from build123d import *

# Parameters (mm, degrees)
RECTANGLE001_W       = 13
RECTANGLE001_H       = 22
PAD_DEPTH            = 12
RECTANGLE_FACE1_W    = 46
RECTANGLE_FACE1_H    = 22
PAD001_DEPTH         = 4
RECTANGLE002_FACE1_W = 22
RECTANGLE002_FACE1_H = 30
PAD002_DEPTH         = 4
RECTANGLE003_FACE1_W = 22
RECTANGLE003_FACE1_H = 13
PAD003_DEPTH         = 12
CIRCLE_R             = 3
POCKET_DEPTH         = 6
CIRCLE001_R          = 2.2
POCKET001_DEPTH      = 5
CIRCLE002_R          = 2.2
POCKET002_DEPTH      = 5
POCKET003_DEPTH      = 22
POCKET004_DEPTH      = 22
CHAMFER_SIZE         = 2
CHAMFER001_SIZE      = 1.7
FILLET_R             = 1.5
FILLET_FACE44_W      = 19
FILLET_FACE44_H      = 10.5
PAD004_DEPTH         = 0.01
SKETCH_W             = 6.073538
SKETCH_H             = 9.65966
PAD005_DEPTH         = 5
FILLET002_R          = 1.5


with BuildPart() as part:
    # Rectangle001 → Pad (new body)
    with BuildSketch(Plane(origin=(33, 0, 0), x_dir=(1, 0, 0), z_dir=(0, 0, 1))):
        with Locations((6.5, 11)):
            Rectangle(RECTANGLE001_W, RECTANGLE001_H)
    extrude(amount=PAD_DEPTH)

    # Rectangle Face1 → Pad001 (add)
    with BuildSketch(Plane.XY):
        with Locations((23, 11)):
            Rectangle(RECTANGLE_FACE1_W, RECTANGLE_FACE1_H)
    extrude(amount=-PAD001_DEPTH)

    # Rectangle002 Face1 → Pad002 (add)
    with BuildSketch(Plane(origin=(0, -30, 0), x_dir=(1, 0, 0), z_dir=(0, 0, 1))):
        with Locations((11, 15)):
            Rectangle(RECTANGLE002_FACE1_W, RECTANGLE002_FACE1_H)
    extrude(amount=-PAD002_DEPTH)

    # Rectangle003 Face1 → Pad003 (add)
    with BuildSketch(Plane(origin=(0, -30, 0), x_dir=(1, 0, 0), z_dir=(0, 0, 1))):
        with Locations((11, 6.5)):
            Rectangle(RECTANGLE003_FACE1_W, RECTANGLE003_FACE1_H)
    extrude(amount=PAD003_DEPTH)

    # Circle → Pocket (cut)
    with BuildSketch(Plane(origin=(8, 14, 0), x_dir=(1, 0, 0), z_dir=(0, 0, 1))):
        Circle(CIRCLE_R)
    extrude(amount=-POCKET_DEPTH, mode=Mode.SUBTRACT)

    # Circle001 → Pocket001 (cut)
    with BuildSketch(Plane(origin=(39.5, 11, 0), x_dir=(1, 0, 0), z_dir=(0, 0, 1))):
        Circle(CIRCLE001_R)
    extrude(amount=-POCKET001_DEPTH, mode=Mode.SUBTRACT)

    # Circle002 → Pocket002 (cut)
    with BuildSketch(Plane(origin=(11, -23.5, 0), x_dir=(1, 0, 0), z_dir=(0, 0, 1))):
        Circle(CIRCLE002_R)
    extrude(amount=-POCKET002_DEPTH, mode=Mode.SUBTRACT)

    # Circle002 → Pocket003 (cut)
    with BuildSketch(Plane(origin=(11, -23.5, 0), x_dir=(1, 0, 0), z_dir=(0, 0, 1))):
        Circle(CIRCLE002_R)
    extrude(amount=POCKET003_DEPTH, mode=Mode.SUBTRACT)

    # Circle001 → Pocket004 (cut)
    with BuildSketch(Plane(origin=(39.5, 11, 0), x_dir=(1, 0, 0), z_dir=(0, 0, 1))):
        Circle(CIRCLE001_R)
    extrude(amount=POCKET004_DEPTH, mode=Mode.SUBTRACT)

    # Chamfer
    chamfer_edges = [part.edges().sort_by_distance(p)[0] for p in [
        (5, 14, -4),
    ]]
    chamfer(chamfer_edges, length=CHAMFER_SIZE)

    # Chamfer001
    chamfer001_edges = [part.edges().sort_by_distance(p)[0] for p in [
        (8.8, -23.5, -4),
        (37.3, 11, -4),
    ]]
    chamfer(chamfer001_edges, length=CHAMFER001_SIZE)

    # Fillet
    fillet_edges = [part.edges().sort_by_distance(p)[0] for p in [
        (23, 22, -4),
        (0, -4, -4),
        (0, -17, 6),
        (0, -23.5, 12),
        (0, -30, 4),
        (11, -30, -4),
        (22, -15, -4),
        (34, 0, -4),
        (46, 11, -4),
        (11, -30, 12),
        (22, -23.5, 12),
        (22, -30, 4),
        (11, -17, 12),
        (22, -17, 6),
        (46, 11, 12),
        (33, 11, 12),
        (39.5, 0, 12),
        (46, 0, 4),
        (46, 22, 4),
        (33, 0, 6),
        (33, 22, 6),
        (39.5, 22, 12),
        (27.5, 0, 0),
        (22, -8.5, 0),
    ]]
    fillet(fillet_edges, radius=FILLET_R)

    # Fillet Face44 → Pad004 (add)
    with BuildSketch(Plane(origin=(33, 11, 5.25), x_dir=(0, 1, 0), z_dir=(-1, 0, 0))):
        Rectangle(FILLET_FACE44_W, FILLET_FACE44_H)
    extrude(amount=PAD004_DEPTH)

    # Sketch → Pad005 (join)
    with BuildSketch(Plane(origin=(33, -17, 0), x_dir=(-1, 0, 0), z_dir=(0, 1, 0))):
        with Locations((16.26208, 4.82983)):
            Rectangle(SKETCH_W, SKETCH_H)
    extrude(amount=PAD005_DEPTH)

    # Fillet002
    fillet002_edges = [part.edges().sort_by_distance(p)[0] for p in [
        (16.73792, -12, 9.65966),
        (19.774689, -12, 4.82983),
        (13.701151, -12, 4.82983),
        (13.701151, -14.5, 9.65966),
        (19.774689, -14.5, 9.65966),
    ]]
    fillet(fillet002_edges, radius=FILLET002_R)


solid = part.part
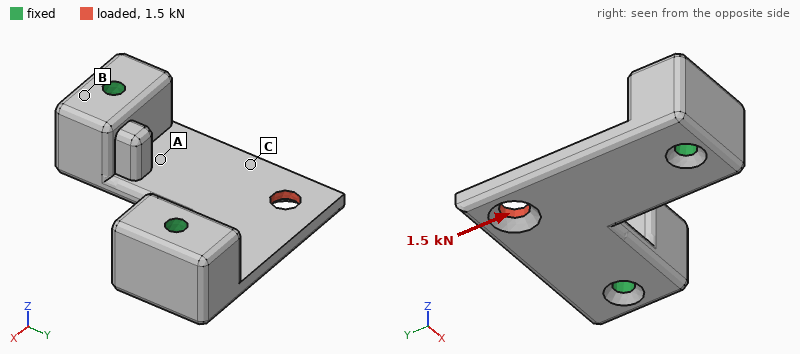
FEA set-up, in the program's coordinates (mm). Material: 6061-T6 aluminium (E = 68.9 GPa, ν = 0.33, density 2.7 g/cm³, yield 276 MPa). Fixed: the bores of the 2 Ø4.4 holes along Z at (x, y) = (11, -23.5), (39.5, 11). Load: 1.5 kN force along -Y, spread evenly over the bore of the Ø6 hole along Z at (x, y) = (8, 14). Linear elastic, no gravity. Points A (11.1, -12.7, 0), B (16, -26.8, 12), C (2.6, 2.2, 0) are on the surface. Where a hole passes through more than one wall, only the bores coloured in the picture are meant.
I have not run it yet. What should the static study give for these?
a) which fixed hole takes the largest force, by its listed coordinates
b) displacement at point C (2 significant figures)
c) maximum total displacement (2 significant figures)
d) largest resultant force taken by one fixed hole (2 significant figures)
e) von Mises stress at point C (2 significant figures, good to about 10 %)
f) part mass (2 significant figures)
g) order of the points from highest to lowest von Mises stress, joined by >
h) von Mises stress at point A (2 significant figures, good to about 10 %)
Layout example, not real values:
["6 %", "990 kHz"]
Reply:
["(11, -23.5)", "10 µm", "44 µm", "1.4 kN", "38 MPa", "35 g", "C > A > B", "23 MPa"]
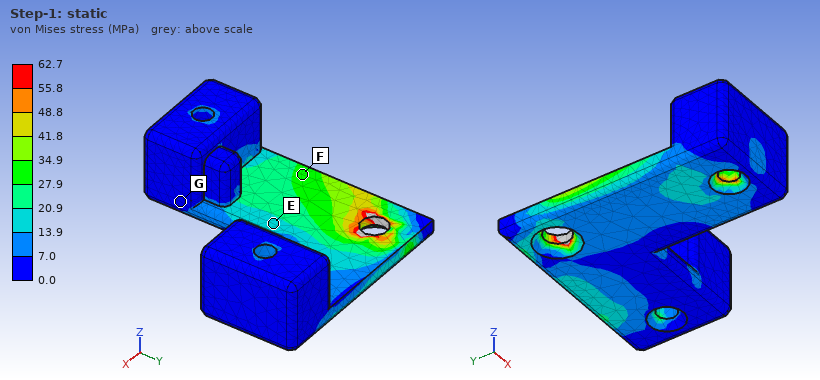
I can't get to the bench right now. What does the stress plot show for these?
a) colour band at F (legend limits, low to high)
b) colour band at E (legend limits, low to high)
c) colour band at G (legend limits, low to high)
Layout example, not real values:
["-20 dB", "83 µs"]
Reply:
["27.9 to 34.9 MPa", "13.9 to 20.9 MPa", "0.0 to 7.0 MPa"]
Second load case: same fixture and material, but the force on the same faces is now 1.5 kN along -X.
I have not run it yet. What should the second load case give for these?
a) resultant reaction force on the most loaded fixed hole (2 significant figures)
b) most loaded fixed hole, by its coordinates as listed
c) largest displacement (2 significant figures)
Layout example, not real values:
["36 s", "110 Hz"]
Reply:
["1.5 kN", "(39.5, 11)", "48 µm"]
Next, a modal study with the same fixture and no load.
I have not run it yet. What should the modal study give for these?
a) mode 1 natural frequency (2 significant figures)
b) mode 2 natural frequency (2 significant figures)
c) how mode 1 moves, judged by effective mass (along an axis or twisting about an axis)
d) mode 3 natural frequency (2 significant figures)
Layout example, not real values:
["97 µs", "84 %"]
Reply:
["4600 Hz", "14 kHz", "along Z", "17 kHz"]
